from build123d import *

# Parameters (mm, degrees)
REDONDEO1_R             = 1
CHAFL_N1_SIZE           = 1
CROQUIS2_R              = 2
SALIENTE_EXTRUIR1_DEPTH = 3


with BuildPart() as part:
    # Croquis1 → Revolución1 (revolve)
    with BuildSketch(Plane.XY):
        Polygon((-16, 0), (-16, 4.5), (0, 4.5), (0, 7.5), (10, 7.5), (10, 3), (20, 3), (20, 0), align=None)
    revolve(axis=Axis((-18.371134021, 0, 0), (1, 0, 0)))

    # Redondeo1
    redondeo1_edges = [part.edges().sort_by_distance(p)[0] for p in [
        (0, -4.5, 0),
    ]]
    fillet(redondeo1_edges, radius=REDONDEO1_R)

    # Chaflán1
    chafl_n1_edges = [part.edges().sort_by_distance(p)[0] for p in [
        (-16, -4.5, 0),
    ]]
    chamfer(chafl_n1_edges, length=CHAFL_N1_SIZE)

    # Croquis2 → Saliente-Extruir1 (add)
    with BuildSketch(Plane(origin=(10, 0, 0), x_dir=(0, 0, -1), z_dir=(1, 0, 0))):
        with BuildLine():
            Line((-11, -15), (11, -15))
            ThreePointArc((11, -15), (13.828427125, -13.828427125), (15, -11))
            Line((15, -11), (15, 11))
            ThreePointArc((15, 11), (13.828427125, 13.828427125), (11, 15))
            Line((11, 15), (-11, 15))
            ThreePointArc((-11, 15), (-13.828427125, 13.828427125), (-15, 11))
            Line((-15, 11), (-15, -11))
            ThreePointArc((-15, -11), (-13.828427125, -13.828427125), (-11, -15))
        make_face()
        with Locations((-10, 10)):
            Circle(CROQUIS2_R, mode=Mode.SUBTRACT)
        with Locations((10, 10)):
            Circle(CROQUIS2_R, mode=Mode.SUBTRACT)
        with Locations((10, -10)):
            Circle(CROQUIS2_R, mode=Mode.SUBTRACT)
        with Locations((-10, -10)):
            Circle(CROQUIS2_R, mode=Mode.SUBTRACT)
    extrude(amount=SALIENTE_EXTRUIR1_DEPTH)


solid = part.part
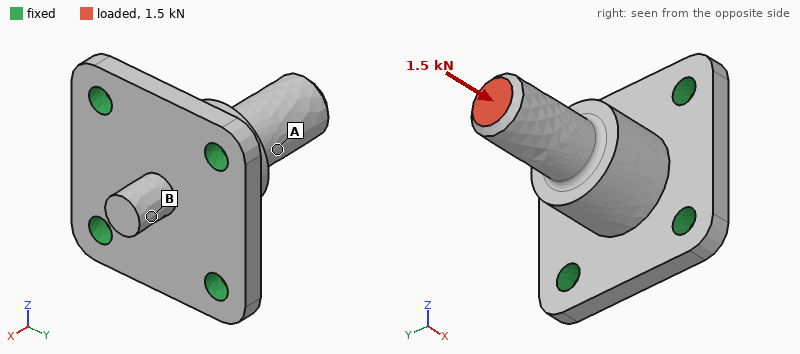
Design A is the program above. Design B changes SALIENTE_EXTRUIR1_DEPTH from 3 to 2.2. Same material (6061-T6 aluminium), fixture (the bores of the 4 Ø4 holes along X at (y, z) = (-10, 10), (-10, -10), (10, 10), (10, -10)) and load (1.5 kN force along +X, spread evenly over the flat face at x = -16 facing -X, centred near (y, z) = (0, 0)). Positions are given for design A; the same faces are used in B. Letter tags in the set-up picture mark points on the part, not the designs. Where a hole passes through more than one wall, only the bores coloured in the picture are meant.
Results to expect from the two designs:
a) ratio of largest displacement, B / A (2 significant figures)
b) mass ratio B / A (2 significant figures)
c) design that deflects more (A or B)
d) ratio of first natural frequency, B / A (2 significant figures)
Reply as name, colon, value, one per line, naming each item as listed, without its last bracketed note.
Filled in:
ratio of largest displacement, B / A: 1.5
mass ratio B / A: 0.88
design that deflects more: B
ratio of first natural frequency, B / A: 0.81
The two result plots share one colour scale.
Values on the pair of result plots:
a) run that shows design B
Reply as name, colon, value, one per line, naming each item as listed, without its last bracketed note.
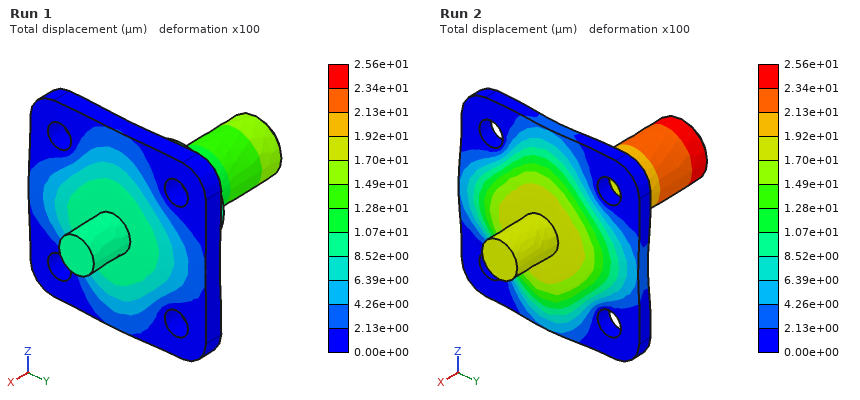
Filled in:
run that shows design B: Run 2
